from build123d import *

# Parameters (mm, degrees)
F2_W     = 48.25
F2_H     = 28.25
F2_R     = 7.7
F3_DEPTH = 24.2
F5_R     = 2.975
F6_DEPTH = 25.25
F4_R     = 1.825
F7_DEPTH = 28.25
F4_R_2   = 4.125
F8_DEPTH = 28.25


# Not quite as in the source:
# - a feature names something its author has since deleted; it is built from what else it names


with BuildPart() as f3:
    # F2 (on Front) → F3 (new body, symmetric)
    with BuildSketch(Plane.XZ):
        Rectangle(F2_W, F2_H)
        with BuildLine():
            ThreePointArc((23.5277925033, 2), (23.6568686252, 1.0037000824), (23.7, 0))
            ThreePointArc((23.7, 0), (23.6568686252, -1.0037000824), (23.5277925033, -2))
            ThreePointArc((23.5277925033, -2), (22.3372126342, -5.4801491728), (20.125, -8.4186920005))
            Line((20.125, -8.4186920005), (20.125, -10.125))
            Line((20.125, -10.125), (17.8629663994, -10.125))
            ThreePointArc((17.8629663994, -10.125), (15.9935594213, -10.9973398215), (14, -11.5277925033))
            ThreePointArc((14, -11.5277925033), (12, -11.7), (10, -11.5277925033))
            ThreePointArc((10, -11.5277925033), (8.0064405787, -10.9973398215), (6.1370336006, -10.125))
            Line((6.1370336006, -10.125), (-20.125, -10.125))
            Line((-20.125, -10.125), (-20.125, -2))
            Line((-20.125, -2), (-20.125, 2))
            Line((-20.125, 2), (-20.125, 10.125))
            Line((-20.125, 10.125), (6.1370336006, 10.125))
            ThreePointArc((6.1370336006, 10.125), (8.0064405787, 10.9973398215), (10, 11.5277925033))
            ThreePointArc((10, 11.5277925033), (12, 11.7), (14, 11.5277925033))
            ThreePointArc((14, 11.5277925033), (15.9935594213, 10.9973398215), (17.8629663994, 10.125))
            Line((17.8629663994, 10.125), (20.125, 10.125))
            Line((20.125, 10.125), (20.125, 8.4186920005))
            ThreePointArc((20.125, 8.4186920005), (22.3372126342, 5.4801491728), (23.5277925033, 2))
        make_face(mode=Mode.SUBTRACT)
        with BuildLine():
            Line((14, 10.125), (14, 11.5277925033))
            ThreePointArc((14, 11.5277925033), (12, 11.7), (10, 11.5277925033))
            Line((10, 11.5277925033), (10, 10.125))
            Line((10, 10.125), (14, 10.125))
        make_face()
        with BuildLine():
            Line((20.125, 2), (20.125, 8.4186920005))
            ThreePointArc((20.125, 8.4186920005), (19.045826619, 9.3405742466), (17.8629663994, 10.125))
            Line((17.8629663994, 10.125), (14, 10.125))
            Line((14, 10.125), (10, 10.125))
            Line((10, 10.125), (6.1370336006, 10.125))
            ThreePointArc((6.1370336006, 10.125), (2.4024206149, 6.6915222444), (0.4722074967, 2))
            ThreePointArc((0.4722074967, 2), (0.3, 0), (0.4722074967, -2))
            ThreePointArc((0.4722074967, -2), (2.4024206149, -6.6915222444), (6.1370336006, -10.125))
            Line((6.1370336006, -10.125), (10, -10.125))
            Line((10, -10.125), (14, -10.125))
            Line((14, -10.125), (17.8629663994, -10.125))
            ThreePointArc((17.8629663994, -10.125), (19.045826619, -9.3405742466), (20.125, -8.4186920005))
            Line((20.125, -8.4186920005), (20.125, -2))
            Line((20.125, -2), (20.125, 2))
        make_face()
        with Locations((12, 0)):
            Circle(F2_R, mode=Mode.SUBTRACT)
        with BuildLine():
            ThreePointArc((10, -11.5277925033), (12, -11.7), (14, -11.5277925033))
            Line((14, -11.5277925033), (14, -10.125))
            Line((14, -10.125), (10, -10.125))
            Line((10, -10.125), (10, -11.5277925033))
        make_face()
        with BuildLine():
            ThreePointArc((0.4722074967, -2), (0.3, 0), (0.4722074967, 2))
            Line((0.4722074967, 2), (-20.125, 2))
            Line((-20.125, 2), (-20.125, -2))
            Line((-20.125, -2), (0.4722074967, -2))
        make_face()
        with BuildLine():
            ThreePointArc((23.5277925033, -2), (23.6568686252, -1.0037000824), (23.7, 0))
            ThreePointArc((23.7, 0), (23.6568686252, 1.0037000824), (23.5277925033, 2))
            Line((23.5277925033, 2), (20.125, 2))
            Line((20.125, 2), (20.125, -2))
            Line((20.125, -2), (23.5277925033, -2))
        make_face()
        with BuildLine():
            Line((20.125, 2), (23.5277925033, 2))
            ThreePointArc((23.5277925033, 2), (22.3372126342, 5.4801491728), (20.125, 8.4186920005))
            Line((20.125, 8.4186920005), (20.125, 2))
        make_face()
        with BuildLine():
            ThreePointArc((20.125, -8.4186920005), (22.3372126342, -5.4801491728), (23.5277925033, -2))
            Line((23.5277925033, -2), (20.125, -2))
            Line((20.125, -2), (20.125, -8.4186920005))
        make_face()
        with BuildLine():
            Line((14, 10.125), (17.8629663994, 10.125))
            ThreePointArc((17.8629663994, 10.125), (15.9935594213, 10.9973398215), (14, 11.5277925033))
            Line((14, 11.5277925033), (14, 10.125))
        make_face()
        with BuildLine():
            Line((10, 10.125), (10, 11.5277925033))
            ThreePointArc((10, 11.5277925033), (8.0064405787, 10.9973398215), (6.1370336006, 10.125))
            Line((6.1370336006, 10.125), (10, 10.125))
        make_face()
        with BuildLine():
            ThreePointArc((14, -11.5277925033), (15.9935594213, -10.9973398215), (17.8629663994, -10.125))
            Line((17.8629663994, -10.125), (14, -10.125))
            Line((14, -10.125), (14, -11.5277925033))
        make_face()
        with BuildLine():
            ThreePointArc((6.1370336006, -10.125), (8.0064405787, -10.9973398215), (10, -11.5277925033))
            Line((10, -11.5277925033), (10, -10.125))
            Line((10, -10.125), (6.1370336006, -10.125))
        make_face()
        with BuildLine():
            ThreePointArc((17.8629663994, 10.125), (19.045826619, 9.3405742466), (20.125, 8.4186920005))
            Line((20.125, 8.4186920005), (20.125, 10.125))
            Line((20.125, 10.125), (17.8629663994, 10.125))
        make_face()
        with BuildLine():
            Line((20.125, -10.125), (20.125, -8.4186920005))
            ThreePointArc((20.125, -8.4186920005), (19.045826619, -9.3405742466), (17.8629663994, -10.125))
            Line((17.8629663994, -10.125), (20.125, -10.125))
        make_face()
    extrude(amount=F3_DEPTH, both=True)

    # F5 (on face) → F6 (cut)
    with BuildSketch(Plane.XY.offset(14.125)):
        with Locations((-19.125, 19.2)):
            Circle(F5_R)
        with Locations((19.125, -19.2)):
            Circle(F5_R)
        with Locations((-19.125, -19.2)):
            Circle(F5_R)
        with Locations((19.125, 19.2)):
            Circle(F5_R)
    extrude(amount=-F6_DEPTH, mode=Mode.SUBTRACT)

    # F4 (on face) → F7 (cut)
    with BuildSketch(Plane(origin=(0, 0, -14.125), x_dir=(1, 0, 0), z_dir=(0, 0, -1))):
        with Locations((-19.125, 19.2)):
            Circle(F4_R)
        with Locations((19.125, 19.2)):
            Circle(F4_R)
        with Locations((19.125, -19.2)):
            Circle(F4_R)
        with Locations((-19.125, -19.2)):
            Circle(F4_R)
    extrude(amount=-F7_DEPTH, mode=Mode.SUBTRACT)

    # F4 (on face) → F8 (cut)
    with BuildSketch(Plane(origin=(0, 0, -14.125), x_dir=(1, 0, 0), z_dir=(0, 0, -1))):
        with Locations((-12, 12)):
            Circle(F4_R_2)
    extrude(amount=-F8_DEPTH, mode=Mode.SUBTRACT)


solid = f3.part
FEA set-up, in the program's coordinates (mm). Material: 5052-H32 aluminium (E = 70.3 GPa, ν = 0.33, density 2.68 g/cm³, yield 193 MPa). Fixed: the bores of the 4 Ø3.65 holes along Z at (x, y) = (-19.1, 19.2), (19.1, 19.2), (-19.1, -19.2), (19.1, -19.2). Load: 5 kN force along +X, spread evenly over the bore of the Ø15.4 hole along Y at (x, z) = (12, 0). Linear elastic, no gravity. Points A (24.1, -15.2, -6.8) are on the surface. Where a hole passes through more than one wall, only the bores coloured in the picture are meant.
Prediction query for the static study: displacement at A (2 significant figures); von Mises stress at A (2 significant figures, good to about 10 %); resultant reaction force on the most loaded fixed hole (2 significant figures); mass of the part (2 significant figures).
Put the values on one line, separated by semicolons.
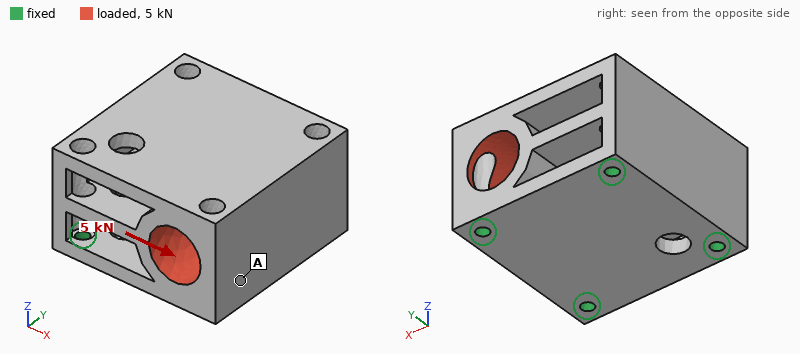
16 µm; 14 MPa; 1.8 kN; 98 g
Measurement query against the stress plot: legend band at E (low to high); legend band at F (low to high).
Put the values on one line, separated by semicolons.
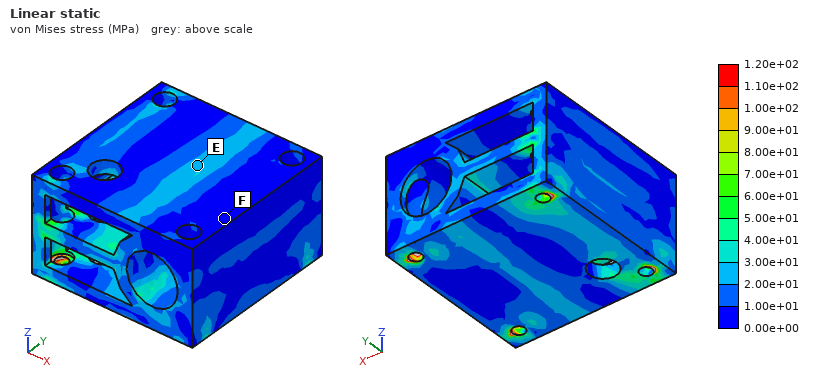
2.00e+01 to 3.00e+01 MPa; 0.00e+00 to 1.00e+01 MPa
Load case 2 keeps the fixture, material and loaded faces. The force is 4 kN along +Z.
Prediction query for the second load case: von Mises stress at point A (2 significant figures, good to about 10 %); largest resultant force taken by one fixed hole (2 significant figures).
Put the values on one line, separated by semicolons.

21 MPa; 1.7 kN
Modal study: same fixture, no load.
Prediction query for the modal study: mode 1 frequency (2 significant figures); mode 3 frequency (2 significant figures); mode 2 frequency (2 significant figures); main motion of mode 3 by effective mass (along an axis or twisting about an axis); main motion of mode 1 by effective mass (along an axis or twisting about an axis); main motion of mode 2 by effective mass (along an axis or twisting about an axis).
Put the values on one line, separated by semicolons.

5600 Hz; 11 kHz; 10 kHz; along Z; along X; along Y
